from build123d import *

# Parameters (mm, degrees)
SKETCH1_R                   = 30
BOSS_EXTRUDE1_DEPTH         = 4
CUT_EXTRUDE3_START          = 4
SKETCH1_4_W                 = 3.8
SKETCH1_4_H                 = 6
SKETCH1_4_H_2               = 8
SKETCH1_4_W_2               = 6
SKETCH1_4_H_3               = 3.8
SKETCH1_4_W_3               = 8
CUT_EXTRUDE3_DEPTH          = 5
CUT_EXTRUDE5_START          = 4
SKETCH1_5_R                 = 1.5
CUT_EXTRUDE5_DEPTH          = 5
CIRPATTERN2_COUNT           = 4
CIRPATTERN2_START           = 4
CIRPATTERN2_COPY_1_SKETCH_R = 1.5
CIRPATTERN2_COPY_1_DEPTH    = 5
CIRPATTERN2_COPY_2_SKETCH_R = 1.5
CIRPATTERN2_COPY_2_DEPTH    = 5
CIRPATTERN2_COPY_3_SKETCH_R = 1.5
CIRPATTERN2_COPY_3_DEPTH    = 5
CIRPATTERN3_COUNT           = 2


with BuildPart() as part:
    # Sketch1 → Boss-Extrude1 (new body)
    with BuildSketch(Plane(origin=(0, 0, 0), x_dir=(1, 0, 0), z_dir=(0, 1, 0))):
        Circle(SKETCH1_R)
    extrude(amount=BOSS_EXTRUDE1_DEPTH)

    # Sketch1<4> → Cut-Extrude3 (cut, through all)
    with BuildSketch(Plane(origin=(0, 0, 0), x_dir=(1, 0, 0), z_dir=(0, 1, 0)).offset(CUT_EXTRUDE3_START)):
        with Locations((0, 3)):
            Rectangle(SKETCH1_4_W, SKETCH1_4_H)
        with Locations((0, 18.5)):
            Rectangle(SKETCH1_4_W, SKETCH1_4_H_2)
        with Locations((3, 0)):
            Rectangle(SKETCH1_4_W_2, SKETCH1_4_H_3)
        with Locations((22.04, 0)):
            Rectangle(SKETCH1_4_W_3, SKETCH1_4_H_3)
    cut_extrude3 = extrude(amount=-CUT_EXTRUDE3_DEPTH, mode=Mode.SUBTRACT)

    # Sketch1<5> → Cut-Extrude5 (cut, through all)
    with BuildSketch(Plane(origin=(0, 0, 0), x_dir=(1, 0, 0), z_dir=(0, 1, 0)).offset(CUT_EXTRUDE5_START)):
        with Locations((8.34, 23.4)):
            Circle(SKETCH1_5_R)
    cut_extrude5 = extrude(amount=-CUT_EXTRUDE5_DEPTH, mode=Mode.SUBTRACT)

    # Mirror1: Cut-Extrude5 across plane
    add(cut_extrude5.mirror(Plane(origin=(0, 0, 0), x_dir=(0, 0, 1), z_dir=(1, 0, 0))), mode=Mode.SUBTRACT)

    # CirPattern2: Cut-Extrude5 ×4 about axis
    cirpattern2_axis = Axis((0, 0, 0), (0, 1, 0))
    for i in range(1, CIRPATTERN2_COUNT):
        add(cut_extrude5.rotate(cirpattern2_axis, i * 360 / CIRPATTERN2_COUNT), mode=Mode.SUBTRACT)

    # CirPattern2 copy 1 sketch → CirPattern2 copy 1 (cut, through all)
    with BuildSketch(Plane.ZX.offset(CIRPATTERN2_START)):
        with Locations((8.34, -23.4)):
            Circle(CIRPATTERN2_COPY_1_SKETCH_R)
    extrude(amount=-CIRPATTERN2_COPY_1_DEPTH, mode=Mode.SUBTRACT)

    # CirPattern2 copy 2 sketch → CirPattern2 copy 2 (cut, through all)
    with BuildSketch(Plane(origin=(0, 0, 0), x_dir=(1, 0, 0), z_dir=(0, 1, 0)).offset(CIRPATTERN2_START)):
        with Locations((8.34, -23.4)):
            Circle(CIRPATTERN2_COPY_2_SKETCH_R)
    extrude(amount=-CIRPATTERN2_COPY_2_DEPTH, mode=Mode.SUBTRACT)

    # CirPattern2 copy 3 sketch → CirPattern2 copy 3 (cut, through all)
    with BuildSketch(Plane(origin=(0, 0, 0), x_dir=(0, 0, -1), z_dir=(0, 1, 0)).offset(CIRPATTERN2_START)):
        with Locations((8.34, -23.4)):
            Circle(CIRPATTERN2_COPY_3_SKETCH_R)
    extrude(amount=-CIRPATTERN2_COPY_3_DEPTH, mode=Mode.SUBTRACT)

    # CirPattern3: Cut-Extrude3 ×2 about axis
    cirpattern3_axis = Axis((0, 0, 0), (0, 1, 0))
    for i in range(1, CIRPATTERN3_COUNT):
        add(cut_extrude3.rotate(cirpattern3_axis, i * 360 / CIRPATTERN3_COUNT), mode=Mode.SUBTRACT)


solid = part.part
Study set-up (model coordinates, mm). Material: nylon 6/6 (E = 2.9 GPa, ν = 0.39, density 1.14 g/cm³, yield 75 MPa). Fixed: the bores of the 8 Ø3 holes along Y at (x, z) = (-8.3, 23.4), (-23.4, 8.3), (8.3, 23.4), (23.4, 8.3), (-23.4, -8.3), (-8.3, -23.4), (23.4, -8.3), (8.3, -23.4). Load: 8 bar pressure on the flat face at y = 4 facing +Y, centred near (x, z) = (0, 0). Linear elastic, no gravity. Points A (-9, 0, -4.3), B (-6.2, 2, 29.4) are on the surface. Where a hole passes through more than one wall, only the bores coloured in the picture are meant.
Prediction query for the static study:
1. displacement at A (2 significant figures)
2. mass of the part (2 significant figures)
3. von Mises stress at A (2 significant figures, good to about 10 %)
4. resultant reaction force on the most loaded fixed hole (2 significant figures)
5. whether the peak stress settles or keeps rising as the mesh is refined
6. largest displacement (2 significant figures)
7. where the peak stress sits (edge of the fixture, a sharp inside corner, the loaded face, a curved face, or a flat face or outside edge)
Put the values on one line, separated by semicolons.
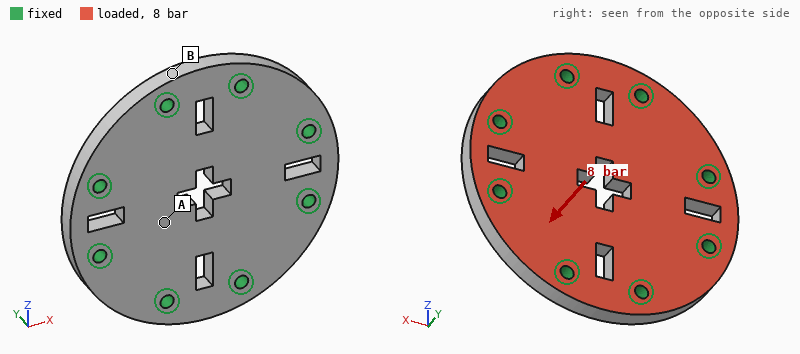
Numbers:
0.28 mm; 12 g; 13 MPa; 260 N; keeps rising; 0.45 mm; edge of the fixture
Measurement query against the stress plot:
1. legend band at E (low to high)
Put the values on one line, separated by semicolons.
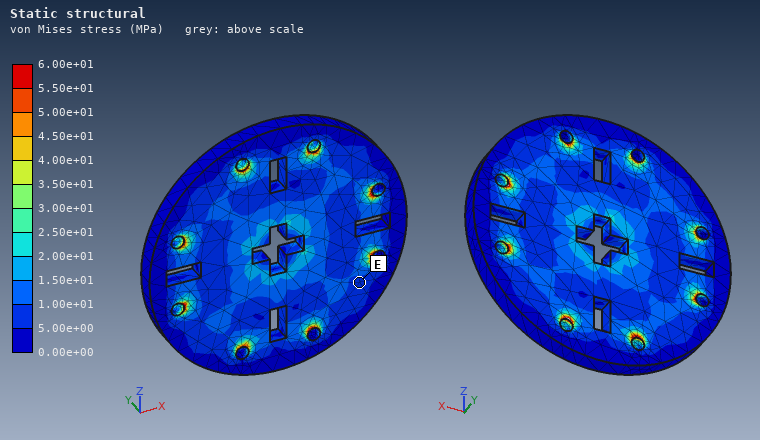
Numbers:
5.00e+00 to 1.00e+01 MPa
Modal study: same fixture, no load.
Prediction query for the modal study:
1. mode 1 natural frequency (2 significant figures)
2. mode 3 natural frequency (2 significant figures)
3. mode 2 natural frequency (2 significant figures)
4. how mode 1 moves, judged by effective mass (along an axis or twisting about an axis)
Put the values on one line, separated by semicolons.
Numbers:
4200 Hz; 7900 Hz; 7900 Hz; along Y
